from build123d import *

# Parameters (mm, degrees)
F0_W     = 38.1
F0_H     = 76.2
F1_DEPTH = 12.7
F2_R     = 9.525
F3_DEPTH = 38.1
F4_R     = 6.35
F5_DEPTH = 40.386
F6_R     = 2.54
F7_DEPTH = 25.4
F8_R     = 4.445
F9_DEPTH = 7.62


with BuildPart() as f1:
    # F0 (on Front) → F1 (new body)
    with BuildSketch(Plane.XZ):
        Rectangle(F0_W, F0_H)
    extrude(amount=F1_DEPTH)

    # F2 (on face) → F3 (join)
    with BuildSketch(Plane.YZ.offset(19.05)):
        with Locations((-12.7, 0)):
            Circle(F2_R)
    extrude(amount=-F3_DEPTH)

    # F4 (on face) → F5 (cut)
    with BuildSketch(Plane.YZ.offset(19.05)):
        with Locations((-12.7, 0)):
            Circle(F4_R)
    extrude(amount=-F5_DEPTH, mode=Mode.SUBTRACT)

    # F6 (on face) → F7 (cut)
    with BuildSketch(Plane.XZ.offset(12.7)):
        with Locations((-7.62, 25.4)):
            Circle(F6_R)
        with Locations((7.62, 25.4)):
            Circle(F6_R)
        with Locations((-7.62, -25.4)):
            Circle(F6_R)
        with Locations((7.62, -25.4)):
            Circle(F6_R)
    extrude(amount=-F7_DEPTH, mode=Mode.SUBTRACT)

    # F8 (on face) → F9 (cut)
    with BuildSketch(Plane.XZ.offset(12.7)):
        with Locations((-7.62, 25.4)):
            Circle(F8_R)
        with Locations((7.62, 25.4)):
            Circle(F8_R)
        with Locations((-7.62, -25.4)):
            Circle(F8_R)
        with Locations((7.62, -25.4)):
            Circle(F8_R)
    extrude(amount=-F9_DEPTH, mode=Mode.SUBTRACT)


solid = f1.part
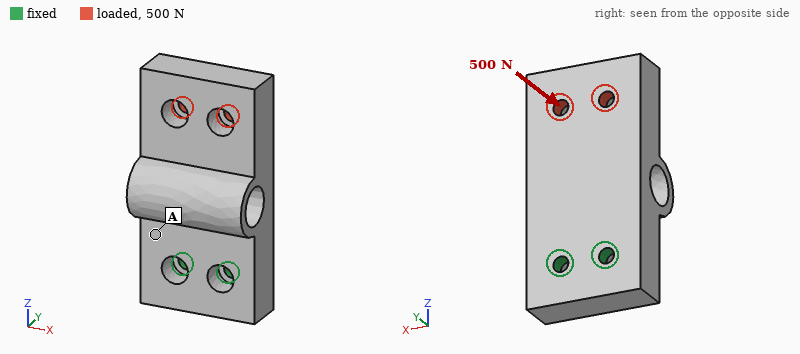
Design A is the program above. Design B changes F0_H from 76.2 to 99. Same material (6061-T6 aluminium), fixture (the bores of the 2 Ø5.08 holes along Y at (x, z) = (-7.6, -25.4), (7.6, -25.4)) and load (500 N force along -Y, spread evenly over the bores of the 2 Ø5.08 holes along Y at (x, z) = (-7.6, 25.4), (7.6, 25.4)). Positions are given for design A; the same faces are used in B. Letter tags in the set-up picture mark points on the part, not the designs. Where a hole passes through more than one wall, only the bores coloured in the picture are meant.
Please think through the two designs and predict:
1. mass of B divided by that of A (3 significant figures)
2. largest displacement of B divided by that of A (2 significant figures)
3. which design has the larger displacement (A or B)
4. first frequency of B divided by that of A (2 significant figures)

1.31
1.2
B
0.74
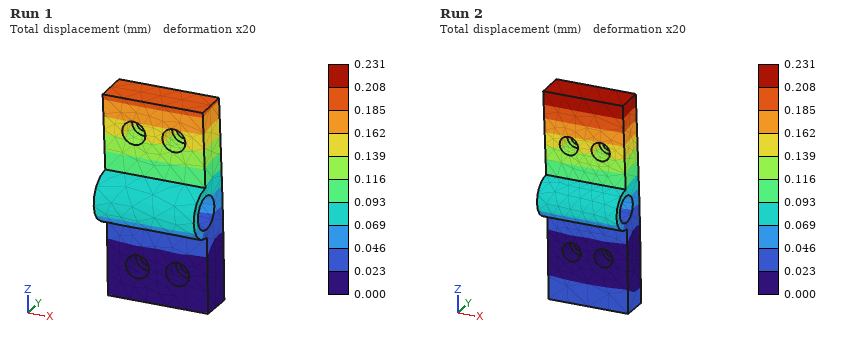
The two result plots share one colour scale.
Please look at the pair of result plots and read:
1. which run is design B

Run 2
